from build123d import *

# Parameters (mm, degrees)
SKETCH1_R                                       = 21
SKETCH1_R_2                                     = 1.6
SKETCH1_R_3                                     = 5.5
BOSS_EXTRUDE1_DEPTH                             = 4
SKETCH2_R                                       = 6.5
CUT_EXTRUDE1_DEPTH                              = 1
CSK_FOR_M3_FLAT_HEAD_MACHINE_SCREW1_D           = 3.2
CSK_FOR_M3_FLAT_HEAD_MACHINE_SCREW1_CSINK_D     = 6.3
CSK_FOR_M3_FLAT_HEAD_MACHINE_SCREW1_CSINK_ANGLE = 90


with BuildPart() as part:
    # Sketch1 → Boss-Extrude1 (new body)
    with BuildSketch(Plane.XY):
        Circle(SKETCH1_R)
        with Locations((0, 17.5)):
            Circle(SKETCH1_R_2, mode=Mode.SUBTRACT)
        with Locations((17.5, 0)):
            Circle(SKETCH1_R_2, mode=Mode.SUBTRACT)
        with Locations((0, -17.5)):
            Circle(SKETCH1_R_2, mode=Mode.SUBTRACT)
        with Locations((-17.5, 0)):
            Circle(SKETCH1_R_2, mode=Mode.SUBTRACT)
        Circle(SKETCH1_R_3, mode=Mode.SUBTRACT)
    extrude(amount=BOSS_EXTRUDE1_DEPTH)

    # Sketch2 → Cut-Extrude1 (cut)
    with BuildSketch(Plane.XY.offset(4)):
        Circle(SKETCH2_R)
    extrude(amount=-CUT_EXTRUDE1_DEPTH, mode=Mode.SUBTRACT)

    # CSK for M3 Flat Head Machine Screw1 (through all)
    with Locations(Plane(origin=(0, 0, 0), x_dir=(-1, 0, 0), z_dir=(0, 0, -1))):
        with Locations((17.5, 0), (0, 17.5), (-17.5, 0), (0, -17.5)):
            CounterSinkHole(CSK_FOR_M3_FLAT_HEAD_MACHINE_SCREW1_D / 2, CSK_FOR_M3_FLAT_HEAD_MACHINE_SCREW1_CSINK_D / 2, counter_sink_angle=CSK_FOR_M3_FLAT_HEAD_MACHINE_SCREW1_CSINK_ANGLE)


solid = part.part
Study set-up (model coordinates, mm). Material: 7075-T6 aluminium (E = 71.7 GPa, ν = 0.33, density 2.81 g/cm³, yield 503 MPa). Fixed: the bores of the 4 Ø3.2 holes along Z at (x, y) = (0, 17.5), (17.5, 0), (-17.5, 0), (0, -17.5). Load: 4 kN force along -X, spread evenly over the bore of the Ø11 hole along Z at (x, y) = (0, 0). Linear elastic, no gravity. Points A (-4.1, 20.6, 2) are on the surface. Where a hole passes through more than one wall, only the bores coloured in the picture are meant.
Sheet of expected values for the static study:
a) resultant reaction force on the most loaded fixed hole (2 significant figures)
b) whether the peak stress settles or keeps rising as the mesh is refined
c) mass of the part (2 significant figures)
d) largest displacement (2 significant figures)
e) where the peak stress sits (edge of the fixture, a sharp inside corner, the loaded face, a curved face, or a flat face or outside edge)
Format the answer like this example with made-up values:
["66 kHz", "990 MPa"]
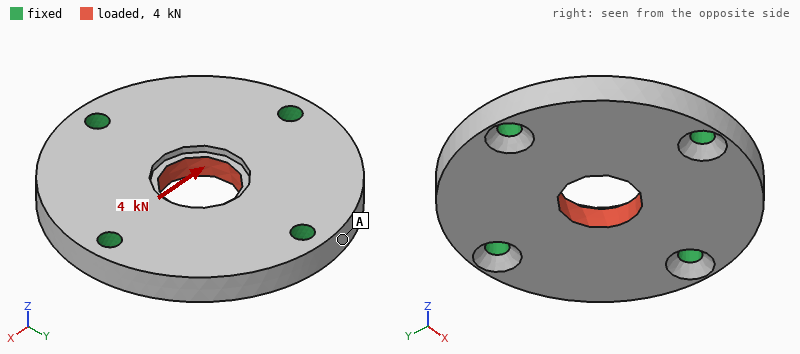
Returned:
["1.3 kN", "keeps rising", "14 g", "8.0 µm", "edge of the fixture"]
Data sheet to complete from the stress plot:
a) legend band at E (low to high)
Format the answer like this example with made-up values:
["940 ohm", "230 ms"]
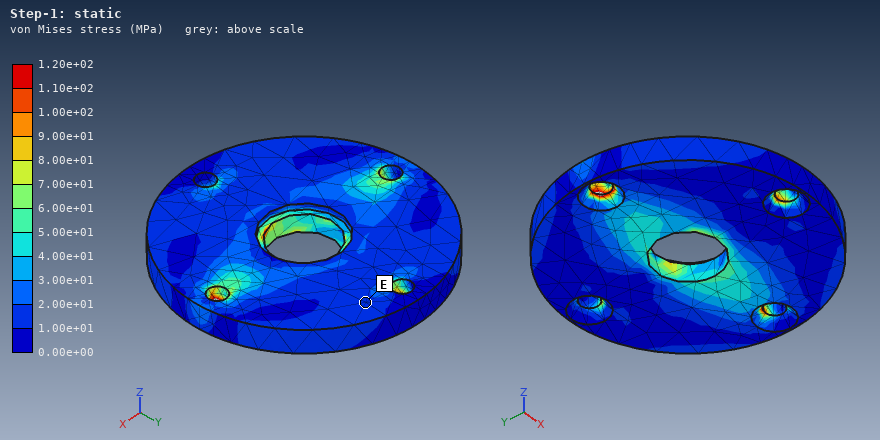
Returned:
["1.00e+01 to 2.00e+01 MPa"]
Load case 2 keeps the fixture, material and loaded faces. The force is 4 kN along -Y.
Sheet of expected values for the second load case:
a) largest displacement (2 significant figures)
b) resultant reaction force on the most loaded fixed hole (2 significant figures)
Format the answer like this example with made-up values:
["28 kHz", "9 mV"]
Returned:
["7.9 µm", "1.3 kN"]
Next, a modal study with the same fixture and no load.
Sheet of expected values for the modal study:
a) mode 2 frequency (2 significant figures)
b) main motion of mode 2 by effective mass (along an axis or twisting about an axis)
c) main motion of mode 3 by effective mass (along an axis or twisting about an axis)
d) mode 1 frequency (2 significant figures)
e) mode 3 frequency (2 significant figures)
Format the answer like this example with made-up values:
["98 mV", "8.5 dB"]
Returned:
["21 kHz", "along Z", "twisting about X", "20 kHz", "22 kHz"]
